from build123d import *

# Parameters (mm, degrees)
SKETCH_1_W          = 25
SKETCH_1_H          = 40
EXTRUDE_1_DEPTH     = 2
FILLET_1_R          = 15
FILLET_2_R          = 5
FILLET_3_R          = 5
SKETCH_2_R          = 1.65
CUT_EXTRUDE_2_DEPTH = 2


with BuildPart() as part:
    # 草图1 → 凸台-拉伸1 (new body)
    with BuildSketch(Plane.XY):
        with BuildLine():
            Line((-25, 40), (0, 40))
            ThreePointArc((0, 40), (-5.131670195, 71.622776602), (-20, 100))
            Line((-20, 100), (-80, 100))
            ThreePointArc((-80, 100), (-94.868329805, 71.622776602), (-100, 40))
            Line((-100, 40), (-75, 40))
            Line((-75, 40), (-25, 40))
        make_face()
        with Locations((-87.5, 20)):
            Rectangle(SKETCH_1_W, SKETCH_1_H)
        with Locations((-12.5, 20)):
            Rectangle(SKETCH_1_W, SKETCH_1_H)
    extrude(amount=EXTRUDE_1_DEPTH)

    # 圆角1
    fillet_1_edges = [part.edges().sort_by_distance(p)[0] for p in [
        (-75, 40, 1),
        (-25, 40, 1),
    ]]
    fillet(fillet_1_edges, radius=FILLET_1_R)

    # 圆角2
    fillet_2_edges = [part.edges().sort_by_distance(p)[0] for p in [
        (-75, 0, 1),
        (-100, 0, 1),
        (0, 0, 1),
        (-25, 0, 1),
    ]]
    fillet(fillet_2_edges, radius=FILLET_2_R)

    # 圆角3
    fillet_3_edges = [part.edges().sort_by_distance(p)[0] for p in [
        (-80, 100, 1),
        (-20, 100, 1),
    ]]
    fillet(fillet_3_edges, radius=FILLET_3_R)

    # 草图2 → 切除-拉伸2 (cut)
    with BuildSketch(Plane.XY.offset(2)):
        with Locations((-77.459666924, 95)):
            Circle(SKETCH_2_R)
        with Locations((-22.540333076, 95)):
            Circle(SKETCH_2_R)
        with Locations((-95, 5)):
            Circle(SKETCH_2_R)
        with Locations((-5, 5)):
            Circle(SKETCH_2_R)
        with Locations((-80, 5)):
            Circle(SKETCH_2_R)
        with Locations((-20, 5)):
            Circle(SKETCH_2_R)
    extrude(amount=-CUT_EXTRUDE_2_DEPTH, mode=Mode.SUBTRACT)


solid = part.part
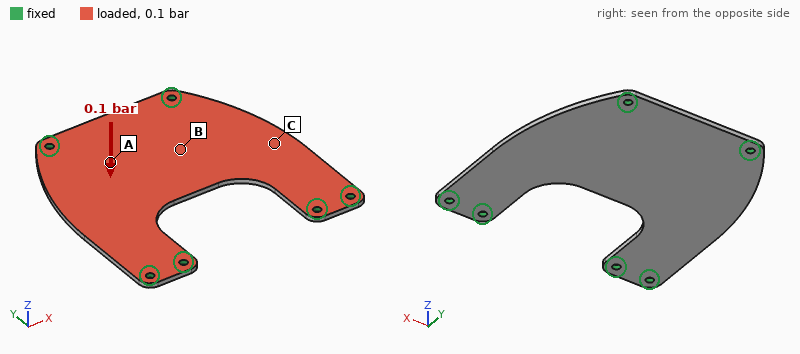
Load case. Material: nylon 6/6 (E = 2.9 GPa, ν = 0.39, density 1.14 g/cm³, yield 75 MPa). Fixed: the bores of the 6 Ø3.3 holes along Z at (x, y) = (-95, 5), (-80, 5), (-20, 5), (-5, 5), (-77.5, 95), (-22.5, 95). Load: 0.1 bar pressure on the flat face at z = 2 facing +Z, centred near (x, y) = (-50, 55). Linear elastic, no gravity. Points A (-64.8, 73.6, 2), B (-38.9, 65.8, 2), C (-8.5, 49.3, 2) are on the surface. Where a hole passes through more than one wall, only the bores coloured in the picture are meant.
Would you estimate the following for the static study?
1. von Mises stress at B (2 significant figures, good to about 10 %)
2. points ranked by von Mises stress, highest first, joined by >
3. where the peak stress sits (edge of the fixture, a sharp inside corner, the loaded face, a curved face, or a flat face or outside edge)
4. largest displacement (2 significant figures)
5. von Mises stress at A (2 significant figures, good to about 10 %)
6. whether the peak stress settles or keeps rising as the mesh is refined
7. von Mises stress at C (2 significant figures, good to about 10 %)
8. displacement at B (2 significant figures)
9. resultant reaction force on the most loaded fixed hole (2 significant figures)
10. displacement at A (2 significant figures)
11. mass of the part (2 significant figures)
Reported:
3.1 MPa
C > B > A
edge of the fixture
1.5 mm
1.8 MPa
keeps rising
5.8 MPa
1.0 mm
20 N
0.75 mm
17 g
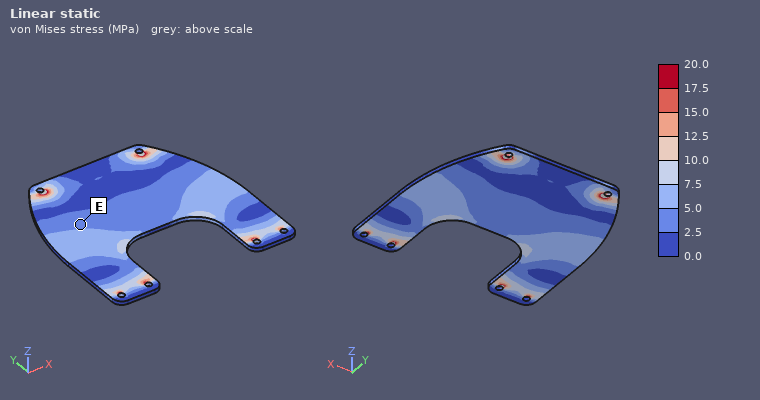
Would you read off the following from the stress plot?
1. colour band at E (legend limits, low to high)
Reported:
2.5 to 5.0 MPa
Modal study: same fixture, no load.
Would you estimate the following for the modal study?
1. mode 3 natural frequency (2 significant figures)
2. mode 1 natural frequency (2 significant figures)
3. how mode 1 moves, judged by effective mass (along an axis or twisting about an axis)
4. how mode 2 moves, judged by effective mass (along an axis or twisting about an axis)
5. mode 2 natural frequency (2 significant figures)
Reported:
590 Hz
330 Hz
along Z
twisting about Y
420 Hz
